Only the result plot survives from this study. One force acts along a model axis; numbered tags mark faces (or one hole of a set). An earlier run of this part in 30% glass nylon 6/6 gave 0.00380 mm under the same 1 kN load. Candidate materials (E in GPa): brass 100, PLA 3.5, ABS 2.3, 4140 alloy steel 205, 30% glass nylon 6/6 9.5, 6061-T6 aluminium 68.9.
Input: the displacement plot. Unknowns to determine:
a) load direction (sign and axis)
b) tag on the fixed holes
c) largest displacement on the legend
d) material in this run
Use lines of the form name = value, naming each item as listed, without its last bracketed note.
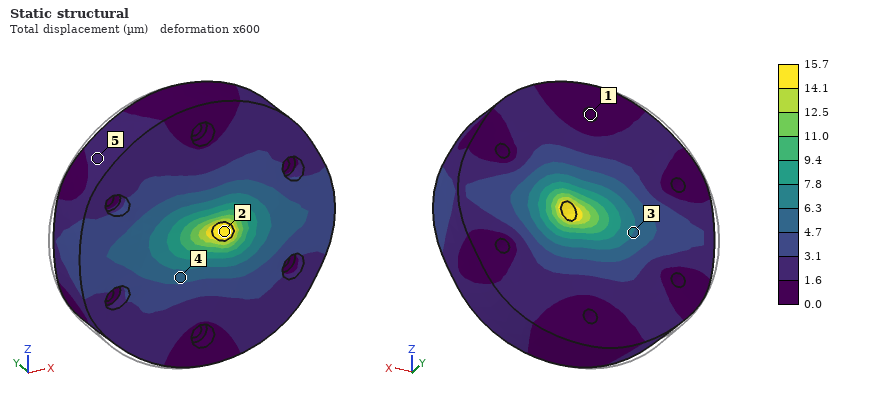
load direction = +X
tag on the fixed holes = 1
largest displacement on the legend = 15.7 µm
material in this run = ABS
